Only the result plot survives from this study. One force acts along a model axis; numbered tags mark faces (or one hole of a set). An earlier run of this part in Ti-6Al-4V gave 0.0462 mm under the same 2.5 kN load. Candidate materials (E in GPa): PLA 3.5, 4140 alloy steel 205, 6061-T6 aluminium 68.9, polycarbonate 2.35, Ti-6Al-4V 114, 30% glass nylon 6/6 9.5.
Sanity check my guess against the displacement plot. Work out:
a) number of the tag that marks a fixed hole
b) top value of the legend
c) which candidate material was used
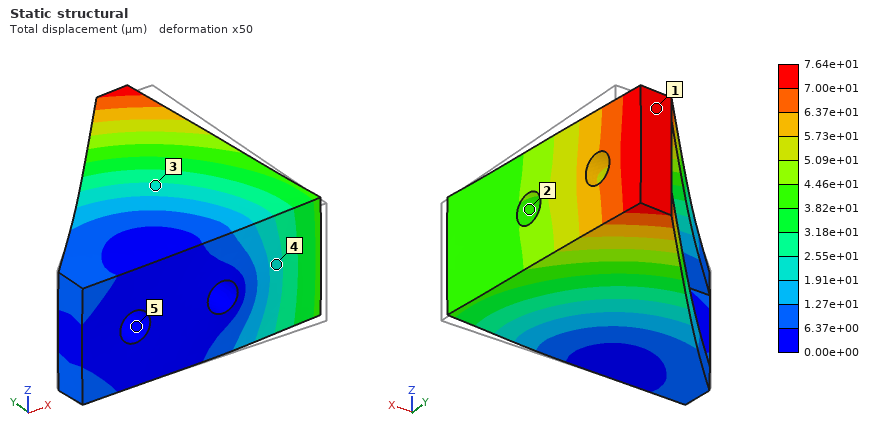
5
7.64e+01 µm
6061-T6 aluminium
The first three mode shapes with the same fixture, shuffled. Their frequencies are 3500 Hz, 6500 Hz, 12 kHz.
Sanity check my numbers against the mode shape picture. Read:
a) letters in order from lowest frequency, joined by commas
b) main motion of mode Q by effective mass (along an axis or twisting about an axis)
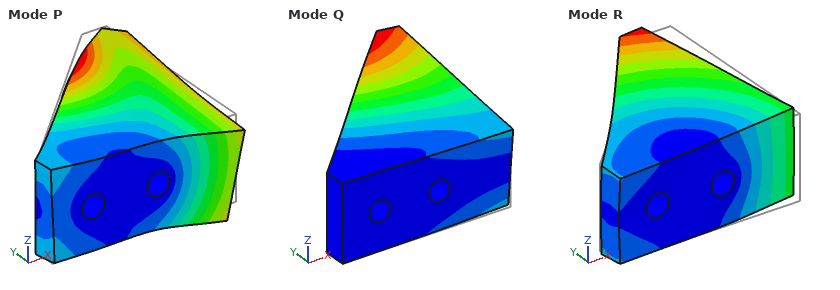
Q, R, P
along Z
